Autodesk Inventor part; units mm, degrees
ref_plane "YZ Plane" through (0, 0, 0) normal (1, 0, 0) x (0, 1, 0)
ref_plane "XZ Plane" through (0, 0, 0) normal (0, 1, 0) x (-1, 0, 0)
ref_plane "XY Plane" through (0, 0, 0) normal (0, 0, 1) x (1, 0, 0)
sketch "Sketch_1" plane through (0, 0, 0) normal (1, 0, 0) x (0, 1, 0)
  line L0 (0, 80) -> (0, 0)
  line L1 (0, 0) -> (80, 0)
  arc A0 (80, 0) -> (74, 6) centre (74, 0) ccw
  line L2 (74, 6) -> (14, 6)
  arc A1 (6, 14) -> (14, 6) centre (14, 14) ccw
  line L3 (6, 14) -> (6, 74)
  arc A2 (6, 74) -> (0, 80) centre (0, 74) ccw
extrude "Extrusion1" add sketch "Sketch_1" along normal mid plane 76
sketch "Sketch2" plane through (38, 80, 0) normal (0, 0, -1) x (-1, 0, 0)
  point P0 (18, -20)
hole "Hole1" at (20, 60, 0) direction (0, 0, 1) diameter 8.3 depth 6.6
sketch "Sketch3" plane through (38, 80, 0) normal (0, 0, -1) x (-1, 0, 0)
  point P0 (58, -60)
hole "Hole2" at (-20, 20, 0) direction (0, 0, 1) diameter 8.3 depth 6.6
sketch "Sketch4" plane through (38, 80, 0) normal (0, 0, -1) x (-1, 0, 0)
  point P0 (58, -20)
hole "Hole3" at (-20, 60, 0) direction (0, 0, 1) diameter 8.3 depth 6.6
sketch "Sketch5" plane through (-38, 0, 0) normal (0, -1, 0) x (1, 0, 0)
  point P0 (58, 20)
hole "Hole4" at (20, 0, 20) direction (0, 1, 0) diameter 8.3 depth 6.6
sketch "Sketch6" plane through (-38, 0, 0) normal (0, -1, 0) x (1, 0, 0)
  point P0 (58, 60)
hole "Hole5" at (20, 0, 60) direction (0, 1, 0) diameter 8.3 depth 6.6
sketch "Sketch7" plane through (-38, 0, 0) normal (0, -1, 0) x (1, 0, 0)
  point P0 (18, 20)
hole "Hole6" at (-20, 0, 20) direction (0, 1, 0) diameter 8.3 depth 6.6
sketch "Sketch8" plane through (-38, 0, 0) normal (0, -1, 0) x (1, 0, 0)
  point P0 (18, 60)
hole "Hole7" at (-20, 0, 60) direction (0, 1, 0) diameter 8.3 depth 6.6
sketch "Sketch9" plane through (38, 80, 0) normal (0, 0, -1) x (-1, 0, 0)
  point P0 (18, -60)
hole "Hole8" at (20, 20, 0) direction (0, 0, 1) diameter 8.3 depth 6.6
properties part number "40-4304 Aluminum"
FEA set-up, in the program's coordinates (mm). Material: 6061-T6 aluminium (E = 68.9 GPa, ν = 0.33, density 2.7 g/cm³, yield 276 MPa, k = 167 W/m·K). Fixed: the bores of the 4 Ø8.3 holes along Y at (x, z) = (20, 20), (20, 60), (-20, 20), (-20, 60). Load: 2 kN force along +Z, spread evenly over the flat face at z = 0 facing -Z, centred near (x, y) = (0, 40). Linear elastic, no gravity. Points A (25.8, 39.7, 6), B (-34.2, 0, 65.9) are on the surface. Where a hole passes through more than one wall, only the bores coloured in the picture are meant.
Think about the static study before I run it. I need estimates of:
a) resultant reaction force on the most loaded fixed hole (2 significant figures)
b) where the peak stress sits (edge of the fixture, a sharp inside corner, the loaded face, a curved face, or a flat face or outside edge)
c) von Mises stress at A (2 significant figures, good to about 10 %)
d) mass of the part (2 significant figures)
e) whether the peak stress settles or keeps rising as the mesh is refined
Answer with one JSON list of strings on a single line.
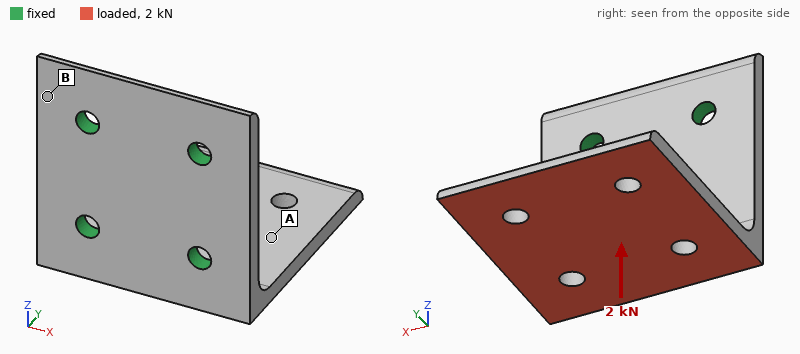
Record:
["920 N", "edge of the fixture", "42 MPa", "180 g", "keeps rising"]
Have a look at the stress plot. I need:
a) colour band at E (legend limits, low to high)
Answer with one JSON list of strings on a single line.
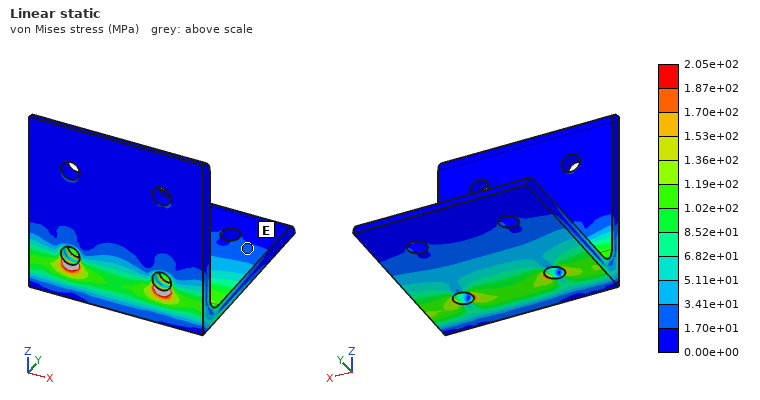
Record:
["1.70e+01 to 3.41e+01 MPa"]
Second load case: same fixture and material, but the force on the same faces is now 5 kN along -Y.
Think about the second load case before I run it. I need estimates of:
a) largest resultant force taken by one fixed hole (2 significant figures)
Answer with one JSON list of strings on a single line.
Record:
["2.7 kN"]
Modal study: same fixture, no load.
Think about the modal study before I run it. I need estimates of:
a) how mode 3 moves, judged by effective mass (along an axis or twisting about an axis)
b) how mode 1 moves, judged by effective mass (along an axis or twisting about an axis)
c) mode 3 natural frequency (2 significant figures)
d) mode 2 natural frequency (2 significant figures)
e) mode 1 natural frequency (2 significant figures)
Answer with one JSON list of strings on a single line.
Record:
["along X", "along Z", "2700 Hz", "1800 Hz", "740 Hz"]
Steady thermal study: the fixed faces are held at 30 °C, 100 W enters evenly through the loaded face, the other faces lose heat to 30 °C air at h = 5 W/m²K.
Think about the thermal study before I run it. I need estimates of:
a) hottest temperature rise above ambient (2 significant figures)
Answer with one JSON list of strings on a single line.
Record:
["67 K"]
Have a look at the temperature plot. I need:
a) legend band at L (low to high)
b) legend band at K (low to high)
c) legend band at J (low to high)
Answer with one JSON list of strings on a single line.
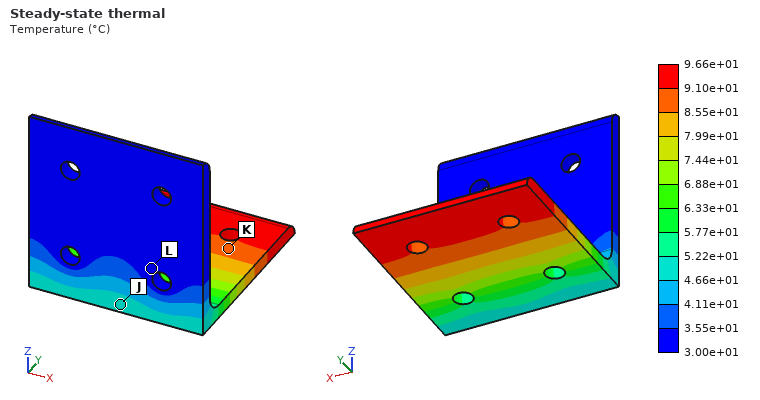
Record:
["3.00e+01 to 3.55e+01 °C", "8.55e+01 to 9.10e+01 °C", "4.66e+01 to 5.22e+01 °C"]
